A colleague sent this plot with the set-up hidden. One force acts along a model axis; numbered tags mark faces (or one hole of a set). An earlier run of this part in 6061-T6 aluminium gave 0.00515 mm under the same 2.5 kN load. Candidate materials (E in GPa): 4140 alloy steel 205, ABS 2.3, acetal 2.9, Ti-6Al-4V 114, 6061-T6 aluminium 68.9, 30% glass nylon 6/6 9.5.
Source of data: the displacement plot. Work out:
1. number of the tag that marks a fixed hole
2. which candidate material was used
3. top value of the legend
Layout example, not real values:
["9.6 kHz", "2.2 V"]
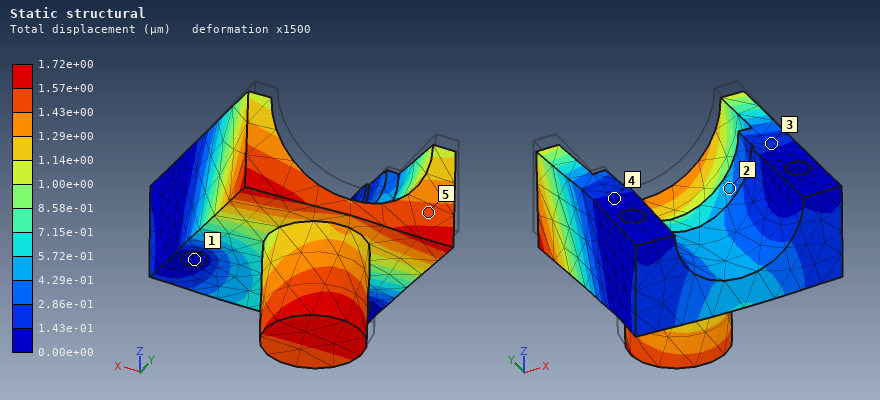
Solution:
["1", "4140 alloy steel", "1.72e+00 µm"]
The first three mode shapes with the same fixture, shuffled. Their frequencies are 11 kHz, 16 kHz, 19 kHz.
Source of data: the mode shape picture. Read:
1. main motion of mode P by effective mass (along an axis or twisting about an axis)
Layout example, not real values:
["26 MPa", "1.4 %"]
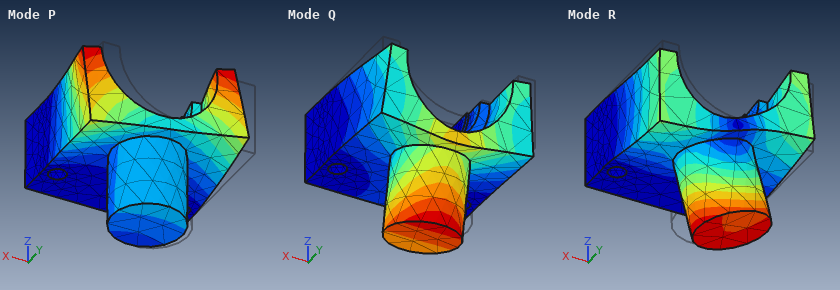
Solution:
["along X"]
